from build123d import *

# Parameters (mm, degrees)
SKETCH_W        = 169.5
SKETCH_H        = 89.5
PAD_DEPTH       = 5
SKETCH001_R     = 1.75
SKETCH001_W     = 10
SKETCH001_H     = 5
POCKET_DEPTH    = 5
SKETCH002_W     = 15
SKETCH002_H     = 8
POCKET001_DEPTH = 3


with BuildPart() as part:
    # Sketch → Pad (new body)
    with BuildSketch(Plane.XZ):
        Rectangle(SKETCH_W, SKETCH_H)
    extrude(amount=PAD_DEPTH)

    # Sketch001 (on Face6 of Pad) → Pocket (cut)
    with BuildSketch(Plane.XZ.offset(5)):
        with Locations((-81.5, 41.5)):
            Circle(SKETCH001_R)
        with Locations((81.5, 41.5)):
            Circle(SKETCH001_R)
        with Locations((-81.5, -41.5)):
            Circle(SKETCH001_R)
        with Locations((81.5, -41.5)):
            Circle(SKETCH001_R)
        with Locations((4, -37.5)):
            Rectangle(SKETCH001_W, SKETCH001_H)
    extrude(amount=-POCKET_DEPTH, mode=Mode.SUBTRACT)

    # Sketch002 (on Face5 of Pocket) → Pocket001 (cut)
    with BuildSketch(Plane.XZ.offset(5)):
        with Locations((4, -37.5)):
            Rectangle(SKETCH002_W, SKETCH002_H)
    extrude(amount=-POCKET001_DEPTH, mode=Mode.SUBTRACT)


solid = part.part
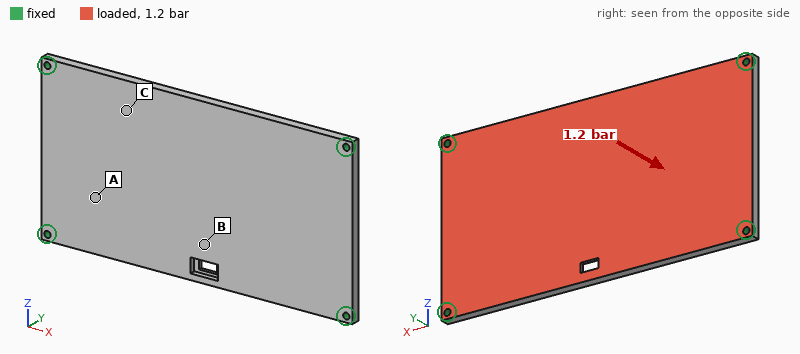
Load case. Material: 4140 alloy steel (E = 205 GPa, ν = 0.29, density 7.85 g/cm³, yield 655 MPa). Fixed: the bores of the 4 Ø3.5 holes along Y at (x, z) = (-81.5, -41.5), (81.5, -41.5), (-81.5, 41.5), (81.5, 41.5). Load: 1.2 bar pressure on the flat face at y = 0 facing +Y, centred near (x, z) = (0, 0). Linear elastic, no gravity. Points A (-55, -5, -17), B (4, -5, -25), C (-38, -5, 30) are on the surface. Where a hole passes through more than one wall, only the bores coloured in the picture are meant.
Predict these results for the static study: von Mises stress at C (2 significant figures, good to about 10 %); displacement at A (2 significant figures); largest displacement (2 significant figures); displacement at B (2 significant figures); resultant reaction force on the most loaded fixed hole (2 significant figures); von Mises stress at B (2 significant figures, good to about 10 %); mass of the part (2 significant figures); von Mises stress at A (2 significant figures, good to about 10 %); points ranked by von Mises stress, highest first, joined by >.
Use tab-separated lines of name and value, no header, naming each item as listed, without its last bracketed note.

von Mises stress at C	26 MPa
displacement at A	0.081 mm
largest displacement	0.19 mm
displacement at B	0.19 mm
resultant reaction force on the most loaded fixed hole	450 N
von Mises stress at B	50 MPa
mass of the part	590 g
von Mises stress at A	14 MPa
points ranked by von Mises stress, highest first, joined by >	B > C > A
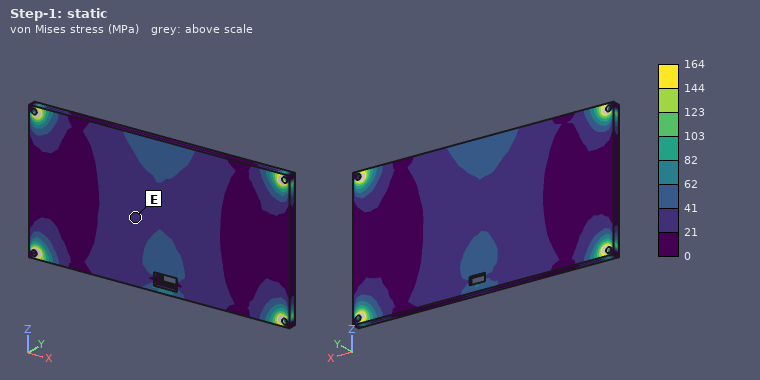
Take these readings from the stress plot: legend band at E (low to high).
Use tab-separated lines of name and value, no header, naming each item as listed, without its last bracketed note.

legend band at E	21 to 41 MPa
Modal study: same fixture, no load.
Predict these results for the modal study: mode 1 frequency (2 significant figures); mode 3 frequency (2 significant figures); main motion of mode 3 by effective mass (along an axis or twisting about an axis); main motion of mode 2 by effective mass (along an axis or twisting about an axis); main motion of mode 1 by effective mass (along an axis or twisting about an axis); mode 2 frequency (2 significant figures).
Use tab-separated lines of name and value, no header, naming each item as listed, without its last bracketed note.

mode 1 frequency	740 Hz
mode 3 frequency	2100 Hz
main motion of mode 3 by effective mass	twisting about Z
main motion of mode 2 by effective mass	twisting about X
main motion of mode 1 by effective mass	along Y
mode 2 frequency	1500 Hz
